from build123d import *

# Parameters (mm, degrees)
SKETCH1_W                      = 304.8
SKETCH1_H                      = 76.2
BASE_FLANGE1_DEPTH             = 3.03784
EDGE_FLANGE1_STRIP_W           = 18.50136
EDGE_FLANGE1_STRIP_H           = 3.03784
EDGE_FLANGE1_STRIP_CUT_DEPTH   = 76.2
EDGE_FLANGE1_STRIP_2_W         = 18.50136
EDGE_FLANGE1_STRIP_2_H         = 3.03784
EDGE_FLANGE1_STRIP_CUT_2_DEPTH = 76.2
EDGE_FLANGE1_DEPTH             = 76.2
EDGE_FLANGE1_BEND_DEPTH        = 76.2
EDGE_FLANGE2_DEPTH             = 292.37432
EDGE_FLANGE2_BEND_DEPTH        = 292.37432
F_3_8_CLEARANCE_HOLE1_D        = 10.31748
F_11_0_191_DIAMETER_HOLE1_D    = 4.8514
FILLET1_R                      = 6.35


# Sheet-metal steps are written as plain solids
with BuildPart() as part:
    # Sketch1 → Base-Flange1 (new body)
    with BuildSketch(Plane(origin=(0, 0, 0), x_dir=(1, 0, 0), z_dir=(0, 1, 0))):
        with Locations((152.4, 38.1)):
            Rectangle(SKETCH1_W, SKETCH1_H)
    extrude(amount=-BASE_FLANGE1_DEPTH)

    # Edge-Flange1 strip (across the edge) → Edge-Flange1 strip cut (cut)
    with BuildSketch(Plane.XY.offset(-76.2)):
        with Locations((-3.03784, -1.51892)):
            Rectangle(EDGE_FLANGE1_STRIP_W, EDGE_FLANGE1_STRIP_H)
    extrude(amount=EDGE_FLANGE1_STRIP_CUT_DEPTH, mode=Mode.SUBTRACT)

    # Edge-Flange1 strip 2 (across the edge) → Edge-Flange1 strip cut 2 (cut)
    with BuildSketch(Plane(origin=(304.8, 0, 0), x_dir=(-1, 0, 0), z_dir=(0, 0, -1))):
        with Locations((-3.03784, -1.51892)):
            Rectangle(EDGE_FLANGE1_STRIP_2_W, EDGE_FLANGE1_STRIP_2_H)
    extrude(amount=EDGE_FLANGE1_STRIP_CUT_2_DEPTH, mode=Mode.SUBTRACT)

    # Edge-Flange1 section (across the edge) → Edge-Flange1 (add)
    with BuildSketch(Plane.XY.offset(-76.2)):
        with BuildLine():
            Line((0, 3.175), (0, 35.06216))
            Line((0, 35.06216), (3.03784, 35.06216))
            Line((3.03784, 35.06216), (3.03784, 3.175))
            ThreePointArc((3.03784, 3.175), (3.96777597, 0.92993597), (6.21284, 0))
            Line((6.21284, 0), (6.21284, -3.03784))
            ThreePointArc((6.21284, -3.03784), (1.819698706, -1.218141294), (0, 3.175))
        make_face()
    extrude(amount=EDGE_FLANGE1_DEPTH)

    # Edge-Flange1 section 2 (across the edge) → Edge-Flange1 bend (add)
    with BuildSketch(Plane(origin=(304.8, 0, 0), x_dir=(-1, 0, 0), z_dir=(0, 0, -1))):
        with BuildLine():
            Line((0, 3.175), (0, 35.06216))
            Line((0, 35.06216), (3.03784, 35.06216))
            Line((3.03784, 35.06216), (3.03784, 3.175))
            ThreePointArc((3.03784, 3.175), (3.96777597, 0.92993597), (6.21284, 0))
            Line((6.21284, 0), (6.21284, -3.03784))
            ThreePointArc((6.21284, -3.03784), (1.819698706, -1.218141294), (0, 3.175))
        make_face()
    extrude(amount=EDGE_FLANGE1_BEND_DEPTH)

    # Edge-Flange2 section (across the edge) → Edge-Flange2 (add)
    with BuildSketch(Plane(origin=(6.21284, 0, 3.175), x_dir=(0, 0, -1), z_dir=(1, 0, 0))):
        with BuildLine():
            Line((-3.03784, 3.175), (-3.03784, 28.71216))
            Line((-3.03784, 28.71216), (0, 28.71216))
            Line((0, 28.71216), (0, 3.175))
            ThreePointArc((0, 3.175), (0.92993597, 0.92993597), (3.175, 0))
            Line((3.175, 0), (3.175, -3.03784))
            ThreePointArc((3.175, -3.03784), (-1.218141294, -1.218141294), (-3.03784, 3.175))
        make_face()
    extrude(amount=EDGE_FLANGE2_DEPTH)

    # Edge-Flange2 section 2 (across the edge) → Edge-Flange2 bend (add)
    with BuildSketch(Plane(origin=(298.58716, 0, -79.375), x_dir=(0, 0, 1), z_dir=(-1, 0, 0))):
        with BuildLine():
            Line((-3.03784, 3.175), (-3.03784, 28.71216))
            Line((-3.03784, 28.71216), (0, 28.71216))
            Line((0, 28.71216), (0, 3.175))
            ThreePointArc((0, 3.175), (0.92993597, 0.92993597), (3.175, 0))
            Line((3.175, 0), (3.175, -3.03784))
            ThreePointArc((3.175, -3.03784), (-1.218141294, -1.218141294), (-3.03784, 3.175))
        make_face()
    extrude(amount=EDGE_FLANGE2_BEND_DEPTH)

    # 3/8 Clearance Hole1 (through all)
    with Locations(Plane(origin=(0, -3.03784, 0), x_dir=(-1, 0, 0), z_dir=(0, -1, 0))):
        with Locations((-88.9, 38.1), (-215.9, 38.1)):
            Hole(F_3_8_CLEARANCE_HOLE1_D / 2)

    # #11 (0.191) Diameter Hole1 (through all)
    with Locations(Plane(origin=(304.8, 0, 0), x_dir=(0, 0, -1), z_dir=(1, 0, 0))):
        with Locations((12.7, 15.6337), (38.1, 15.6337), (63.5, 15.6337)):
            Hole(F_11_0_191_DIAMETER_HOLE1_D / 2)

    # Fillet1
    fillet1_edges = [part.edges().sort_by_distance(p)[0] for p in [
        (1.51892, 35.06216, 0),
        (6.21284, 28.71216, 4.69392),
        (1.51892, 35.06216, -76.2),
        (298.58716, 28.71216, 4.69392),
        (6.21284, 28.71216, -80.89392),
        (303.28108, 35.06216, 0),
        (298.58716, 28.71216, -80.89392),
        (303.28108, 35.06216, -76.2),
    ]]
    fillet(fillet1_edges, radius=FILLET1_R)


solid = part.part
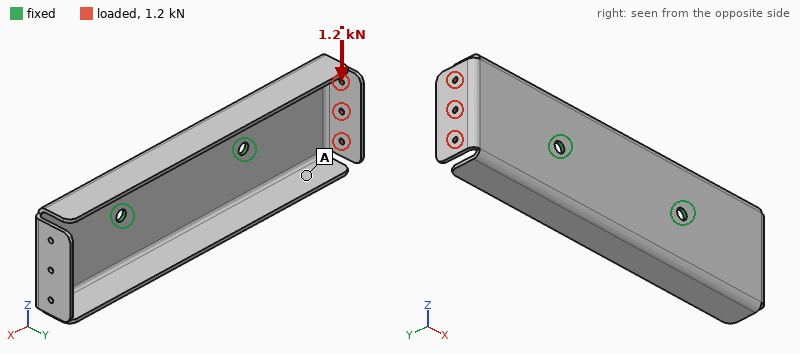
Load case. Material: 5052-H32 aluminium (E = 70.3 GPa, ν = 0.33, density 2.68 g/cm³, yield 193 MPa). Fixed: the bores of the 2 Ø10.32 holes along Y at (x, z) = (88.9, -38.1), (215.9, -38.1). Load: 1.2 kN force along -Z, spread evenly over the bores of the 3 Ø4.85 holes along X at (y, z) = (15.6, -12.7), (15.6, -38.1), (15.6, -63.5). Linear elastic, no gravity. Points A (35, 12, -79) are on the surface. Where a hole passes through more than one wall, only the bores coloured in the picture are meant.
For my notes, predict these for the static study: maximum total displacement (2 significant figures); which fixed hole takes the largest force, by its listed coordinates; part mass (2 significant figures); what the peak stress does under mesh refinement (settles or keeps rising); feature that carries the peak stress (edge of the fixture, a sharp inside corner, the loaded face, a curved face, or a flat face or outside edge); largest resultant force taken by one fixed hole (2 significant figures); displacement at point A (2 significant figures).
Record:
1.7 mm
(88.9, -38.1)
380 g
keeps rising
edge of the fixture
1.9 kN
1.1 mm
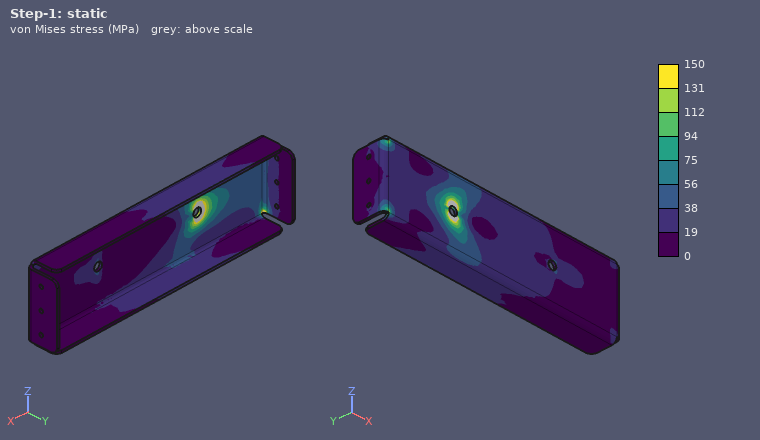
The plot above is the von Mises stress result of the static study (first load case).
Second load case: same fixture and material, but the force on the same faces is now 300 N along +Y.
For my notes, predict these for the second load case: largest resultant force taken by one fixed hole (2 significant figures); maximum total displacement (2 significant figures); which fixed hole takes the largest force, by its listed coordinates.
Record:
570 N
0.58 mm
(88.9, -38.1)
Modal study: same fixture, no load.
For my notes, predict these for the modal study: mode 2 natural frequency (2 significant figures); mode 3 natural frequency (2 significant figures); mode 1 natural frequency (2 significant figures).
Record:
400 Hz
410 Hz
380 Hz
